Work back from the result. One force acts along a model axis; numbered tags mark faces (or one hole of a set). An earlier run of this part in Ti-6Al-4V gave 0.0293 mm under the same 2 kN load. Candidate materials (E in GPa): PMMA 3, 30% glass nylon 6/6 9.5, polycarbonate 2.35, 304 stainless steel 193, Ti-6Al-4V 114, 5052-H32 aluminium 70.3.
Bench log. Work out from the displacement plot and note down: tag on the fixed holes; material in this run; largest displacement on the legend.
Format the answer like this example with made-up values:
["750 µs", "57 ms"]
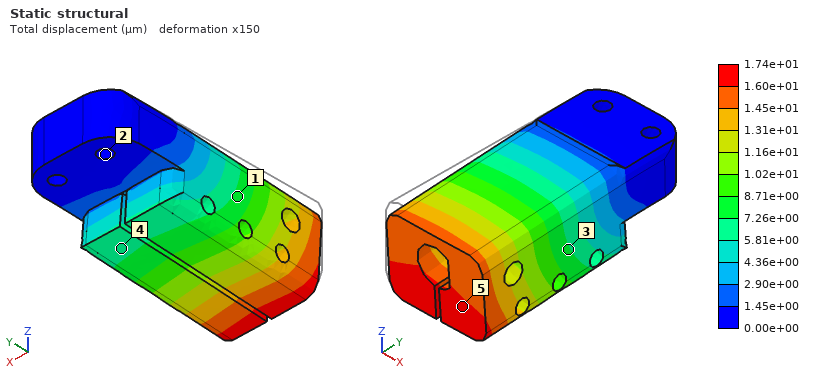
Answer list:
["2", "304 stainless steel", "1.74e+01 µm"]
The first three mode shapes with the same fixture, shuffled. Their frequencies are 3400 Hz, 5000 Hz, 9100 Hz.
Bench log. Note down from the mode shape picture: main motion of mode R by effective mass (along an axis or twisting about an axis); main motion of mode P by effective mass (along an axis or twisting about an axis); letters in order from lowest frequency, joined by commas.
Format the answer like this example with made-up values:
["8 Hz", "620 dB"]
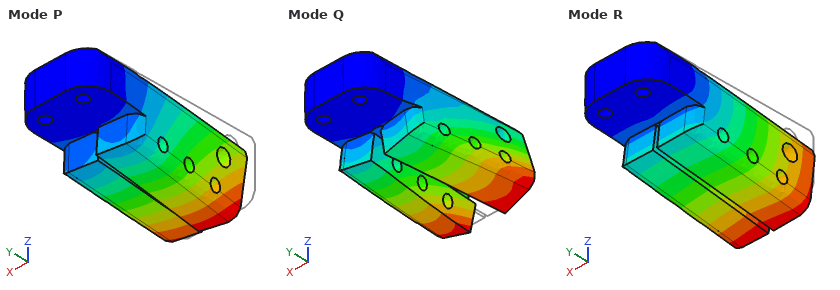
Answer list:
["along Z", "along X", "R, P, Q"]
